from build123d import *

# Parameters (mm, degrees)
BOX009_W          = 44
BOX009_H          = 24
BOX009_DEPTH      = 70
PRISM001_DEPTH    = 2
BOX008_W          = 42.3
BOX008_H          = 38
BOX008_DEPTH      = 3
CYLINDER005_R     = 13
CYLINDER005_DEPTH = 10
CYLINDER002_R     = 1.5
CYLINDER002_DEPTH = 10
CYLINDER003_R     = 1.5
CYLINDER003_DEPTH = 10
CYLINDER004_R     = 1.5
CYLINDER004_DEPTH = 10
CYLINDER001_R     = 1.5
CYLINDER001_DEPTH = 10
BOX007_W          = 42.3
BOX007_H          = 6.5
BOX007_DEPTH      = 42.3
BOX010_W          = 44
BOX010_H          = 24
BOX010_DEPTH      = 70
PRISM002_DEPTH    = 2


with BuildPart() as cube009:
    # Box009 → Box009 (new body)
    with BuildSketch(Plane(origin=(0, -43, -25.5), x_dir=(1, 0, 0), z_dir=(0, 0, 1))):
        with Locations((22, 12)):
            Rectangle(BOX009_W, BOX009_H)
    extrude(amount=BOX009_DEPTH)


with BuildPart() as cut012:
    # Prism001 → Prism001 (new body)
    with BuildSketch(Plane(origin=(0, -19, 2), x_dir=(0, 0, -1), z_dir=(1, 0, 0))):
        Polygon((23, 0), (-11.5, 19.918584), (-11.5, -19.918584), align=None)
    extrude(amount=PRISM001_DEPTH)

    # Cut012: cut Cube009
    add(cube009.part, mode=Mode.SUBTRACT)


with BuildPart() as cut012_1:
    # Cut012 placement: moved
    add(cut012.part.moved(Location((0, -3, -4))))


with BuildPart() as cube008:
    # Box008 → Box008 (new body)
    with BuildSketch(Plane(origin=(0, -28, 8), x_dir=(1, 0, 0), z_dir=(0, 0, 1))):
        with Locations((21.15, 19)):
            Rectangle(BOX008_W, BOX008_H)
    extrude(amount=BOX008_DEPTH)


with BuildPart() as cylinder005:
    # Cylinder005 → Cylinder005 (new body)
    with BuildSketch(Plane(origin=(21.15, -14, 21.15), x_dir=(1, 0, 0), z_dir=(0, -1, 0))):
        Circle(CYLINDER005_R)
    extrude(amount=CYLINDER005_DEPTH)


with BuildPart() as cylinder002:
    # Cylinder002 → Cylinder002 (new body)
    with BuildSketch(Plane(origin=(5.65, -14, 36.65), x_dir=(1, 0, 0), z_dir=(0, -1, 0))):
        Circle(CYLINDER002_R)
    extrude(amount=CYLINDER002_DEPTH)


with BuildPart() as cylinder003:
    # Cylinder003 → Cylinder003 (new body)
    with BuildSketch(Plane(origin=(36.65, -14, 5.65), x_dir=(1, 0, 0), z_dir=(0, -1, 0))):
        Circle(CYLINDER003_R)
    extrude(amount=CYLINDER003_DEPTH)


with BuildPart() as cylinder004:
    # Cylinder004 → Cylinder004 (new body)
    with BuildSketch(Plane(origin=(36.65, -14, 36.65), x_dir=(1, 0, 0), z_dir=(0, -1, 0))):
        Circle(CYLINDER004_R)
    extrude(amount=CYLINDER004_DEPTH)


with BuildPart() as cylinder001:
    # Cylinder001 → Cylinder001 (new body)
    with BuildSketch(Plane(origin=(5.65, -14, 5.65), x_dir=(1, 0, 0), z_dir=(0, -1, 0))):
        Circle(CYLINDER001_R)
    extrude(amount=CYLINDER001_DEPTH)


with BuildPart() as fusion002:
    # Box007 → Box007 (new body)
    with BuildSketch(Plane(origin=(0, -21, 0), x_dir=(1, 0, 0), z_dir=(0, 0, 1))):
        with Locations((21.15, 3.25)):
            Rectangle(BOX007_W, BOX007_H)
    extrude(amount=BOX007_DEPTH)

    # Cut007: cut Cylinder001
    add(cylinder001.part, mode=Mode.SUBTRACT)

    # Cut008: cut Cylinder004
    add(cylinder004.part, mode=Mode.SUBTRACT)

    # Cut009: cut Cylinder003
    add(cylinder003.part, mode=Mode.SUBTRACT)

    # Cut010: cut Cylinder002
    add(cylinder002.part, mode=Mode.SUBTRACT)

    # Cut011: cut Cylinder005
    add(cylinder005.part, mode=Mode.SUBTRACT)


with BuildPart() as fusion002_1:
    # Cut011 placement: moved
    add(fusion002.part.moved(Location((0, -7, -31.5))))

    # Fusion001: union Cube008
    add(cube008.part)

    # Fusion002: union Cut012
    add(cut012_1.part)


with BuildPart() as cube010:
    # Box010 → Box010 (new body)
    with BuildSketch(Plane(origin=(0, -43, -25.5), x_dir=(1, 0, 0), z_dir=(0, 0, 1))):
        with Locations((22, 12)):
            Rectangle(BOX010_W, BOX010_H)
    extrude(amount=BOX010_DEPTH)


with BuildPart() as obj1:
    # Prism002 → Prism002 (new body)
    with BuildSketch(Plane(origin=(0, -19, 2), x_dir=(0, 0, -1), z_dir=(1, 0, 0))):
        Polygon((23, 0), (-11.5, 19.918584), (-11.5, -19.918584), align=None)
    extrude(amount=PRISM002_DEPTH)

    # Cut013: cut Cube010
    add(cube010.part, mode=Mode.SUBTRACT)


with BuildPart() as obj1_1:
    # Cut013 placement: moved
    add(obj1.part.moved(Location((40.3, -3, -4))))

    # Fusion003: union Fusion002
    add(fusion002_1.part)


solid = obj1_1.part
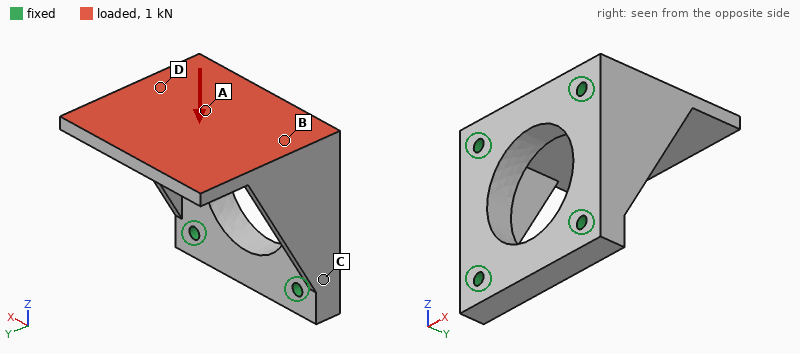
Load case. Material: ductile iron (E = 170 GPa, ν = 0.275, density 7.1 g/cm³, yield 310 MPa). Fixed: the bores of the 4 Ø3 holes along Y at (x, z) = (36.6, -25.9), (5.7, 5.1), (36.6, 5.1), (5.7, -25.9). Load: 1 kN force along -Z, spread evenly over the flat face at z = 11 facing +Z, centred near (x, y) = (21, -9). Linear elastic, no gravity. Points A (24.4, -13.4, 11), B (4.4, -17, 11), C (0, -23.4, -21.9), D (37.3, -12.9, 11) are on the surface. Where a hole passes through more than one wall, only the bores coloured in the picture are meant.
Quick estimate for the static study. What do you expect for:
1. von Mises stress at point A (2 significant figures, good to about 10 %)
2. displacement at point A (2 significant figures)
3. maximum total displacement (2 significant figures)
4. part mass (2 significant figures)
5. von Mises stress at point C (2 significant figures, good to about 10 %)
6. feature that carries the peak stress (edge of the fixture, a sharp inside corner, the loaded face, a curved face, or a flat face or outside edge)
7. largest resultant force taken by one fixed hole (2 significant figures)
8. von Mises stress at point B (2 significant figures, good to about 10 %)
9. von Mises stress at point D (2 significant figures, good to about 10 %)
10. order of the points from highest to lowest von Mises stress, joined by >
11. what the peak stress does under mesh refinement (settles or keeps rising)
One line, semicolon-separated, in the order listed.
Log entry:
29 MPa; 14 µm; 77 µm; 94 g; 14 MPa; a sharp inside corner; 420 N; 39 MPa; 47 MPa; D > B > A > C; keeps rising
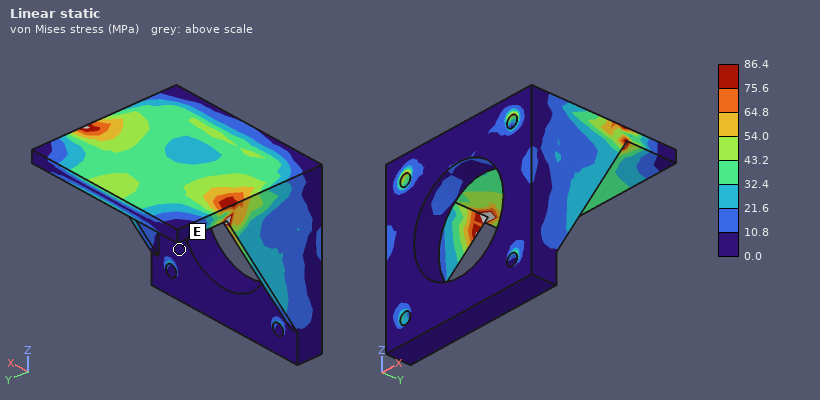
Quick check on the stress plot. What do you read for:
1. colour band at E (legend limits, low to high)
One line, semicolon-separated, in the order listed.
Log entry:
0.0 to 10.8 MPa
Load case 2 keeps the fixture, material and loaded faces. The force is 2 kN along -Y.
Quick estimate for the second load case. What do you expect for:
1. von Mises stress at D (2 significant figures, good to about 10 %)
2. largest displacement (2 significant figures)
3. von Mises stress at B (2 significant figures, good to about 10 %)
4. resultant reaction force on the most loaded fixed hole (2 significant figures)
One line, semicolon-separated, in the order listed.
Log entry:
25 MPa; 29 µm; 23 MPa; 1.1 kN
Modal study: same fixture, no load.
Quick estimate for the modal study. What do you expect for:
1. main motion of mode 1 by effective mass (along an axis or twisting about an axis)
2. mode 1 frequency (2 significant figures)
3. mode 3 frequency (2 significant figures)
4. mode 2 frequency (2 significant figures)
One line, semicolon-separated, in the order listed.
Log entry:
along Z; 4100 Hz; 13 kHz; 8900 Hz
